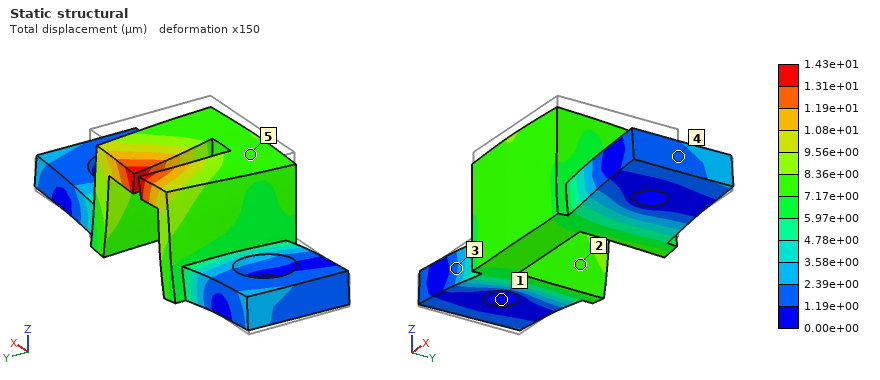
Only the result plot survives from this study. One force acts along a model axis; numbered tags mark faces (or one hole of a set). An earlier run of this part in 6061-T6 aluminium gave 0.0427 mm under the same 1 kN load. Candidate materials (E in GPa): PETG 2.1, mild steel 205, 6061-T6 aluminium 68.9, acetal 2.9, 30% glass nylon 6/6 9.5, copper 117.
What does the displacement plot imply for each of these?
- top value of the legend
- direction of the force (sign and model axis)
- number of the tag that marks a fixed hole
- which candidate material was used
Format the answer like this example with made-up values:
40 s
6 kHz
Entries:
1.43e+01 µm
-Z
1
mild steel
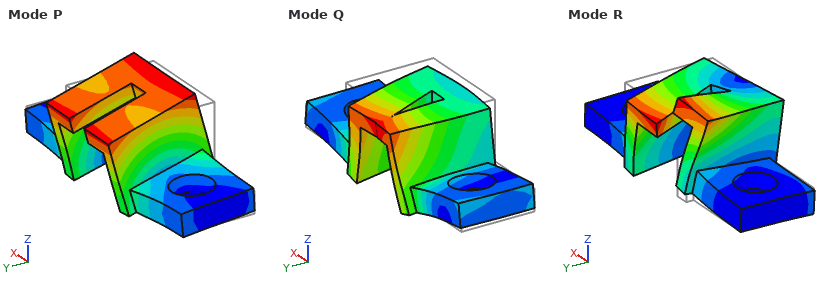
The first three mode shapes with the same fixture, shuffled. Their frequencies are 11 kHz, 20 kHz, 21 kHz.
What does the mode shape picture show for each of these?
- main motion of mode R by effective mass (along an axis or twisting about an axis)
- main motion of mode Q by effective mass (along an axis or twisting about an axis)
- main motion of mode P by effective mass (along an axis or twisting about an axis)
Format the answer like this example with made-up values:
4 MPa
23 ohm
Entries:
along X
along Z
along Y
